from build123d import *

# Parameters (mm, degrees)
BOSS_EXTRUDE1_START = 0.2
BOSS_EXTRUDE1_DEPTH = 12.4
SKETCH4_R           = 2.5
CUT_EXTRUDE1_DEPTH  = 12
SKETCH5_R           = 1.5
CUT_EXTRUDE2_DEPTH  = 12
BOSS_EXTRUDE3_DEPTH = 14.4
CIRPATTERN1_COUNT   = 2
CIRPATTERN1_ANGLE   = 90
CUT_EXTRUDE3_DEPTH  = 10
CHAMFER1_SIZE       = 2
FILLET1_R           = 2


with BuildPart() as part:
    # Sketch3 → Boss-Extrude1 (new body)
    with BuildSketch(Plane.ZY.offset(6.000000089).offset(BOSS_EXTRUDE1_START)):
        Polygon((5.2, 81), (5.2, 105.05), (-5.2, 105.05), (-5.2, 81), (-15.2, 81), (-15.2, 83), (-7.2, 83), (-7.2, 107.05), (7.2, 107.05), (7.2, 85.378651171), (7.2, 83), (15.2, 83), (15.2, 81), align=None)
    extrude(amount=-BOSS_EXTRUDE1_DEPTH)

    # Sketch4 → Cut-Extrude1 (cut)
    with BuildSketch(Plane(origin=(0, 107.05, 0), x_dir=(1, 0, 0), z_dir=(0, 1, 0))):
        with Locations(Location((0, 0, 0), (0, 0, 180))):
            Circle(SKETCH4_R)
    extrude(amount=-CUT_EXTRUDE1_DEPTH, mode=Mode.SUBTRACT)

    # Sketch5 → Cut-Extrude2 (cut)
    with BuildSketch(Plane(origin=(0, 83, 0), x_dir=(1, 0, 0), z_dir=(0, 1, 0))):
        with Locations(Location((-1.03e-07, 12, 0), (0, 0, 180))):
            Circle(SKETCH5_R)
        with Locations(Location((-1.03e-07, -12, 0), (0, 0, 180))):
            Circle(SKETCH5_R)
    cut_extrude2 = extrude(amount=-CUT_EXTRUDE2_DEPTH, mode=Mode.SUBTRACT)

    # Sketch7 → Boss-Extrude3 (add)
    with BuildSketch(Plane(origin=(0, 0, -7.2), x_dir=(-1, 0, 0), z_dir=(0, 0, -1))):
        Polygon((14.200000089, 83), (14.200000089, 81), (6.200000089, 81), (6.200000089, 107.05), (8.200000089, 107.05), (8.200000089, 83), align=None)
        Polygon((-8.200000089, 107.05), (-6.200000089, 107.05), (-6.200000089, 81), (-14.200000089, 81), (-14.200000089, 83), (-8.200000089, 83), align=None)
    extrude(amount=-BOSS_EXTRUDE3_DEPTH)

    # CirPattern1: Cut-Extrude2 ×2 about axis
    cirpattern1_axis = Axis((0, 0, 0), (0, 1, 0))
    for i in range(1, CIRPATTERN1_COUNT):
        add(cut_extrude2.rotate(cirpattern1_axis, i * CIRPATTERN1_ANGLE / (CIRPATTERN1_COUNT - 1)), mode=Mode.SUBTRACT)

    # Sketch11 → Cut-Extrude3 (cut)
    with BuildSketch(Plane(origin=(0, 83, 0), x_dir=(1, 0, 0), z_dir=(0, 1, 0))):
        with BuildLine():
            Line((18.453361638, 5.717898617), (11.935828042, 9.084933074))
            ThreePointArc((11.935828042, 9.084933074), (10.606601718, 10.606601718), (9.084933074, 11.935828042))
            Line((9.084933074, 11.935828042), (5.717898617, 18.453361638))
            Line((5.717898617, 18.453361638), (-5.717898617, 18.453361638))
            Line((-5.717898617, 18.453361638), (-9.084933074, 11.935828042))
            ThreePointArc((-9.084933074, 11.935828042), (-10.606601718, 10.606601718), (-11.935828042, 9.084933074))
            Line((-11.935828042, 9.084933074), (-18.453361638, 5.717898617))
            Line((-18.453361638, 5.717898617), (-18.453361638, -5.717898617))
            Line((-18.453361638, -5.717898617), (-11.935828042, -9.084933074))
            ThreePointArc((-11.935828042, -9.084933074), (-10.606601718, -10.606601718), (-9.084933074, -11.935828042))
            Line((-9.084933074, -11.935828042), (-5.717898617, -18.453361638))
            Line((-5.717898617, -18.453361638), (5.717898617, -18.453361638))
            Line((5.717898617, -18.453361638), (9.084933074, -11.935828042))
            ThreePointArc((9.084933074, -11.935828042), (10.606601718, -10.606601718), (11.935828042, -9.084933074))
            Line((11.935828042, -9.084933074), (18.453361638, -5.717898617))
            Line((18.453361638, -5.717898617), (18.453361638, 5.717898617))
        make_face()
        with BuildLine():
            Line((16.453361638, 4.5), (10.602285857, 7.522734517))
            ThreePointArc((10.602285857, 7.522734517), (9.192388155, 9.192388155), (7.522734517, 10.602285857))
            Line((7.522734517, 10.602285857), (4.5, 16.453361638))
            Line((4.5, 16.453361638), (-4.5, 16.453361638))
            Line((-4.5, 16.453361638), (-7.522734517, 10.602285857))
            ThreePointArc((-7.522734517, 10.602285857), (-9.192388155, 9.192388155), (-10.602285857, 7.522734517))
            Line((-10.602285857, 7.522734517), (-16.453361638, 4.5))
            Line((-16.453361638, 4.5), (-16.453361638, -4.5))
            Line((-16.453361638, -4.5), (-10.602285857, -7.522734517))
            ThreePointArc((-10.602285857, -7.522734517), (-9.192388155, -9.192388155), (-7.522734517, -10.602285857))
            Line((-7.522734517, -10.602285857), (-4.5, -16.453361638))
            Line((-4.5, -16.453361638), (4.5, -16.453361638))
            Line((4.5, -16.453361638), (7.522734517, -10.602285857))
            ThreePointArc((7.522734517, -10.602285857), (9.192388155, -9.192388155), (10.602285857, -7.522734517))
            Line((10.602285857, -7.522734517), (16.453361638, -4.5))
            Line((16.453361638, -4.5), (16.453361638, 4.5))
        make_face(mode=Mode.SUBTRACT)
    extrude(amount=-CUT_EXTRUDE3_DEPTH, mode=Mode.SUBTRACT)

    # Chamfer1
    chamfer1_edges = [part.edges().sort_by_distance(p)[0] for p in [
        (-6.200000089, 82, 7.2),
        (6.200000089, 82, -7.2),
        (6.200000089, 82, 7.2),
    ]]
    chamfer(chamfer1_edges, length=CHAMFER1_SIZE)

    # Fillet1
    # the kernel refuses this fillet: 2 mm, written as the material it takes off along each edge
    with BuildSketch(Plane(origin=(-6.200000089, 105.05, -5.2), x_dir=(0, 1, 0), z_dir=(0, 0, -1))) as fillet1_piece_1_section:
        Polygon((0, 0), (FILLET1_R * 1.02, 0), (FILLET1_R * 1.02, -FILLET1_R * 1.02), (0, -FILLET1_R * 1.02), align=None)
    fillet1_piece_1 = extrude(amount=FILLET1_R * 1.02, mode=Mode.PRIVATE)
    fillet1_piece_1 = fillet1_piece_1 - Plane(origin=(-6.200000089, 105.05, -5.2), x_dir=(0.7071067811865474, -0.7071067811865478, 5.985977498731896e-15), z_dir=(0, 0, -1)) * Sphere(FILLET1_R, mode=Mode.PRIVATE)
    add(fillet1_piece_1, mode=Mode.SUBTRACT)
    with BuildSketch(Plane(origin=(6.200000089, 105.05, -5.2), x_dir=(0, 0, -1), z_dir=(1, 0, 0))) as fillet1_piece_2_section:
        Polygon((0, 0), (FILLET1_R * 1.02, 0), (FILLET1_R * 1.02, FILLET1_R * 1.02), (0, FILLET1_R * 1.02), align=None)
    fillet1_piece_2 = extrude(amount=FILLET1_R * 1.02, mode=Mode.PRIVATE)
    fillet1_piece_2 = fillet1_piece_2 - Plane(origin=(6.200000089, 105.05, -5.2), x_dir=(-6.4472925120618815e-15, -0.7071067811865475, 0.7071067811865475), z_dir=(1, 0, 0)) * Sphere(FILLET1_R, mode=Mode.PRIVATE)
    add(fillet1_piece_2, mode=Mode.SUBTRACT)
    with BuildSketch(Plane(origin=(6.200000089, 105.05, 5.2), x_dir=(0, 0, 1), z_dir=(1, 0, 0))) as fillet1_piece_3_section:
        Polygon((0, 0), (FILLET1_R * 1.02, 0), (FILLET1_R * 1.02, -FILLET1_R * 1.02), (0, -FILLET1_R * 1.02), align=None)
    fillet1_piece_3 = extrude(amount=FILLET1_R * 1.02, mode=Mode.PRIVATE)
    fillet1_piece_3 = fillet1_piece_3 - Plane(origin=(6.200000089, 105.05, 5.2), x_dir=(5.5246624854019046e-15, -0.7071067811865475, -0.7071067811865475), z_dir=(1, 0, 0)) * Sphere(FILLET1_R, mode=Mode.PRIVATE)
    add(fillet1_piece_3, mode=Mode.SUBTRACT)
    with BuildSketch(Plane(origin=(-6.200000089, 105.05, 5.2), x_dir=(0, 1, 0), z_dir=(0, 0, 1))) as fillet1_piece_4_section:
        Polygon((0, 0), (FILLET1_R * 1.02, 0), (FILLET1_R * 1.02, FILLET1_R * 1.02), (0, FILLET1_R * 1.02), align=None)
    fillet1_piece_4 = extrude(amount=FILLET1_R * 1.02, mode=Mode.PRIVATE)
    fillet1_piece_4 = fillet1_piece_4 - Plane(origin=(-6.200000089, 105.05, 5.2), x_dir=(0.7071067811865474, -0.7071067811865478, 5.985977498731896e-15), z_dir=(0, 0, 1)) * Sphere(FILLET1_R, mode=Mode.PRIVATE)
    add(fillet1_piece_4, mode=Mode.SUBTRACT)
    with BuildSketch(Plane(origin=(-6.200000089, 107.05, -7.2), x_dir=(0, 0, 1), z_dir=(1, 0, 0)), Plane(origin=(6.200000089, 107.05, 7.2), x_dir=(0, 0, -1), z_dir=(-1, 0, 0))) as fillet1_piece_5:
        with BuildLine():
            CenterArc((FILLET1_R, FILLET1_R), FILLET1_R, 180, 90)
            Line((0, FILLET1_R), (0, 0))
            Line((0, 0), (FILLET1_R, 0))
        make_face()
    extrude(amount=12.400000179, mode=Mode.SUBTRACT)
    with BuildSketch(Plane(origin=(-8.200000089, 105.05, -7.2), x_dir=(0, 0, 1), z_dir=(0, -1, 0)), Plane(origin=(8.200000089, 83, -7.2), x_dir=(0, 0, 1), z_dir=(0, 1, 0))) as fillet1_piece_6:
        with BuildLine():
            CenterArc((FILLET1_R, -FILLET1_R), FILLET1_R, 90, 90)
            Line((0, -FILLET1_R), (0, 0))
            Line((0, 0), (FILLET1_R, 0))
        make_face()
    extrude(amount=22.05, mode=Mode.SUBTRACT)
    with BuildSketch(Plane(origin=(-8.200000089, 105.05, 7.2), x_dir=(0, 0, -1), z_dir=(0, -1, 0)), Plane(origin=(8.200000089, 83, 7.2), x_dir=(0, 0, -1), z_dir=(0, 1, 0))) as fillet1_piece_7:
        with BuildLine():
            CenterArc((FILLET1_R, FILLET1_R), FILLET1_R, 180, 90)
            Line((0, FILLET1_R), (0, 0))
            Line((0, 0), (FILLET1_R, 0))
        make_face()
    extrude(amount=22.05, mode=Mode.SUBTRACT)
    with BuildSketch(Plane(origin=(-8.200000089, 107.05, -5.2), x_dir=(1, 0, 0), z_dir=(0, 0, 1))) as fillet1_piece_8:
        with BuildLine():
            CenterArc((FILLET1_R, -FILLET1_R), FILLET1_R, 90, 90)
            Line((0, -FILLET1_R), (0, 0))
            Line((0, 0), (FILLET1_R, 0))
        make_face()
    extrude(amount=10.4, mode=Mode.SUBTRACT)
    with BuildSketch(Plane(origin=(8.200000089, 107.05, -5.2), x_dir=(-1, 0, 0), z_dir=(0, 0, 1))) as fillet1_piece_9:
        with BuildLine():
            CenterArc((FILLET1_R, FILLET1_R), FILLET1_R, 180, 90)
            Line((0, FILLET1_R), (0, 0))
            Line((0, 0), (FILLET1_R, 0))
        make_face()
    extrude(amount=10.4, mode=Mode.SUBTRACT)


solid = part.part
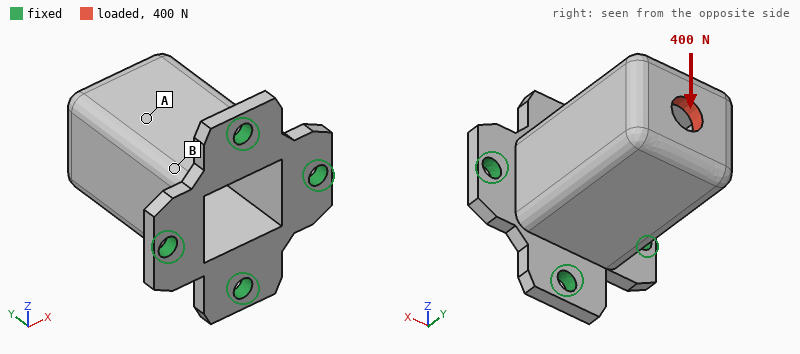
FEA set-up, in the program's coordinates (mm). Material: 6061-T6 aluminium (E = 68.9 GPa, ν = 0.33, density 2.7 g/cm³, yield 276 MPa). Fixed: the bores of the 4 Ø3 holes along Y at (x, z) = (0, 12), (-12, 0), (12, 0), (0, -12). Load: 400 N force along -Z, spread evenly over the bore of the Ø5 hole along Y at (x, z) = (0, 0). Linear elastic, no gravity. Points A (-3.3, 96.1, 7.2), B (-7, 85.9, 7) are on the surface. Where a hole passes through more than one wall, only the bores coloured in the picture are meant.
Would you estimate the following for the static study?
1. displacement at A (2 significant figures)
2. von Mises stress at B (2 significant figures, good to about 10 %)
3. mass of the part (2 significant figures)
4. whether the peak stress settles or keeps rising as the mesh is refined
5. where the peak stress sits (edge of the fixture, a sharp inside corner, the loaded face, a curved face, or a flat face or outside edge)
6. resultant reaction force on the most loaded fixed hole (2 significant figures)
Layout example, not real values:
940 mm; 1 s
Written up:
41 µm; 30 MPa; 9.6 g; keeps rising; edge of the fixture; 490 N
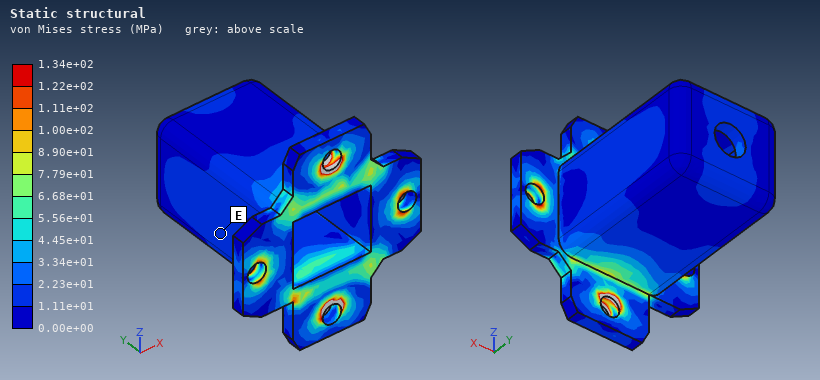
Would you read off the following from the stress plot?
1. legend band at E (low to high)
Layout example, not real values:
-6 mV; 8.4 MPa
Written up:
1.11e+01 to 2.23e+01 MPa
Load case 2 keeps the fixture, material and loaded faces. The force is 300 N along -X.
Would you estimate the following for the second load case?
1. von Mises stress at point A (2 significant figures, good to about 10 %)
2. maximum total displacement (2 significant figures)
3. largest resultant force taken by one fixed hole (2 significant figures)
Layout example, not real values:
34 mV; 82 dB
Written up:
11 MPa; 37 µm; 370 N
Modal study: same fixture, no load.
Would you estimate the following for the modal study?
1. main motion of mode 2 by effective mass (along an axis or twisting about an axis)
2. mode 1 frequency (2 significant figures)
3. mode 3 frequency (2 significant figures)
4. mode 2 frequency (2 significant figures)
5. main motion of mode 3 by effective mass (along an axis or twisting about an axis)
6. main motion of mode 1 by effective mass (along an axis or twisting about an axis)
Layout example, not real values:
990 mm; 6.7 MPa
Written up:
along X; 6900 Hz; 19 kHz; 8400 Hz; along Y; along Z
